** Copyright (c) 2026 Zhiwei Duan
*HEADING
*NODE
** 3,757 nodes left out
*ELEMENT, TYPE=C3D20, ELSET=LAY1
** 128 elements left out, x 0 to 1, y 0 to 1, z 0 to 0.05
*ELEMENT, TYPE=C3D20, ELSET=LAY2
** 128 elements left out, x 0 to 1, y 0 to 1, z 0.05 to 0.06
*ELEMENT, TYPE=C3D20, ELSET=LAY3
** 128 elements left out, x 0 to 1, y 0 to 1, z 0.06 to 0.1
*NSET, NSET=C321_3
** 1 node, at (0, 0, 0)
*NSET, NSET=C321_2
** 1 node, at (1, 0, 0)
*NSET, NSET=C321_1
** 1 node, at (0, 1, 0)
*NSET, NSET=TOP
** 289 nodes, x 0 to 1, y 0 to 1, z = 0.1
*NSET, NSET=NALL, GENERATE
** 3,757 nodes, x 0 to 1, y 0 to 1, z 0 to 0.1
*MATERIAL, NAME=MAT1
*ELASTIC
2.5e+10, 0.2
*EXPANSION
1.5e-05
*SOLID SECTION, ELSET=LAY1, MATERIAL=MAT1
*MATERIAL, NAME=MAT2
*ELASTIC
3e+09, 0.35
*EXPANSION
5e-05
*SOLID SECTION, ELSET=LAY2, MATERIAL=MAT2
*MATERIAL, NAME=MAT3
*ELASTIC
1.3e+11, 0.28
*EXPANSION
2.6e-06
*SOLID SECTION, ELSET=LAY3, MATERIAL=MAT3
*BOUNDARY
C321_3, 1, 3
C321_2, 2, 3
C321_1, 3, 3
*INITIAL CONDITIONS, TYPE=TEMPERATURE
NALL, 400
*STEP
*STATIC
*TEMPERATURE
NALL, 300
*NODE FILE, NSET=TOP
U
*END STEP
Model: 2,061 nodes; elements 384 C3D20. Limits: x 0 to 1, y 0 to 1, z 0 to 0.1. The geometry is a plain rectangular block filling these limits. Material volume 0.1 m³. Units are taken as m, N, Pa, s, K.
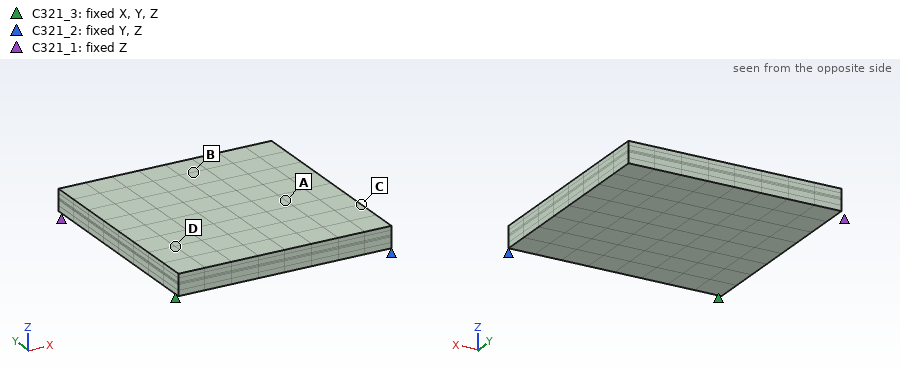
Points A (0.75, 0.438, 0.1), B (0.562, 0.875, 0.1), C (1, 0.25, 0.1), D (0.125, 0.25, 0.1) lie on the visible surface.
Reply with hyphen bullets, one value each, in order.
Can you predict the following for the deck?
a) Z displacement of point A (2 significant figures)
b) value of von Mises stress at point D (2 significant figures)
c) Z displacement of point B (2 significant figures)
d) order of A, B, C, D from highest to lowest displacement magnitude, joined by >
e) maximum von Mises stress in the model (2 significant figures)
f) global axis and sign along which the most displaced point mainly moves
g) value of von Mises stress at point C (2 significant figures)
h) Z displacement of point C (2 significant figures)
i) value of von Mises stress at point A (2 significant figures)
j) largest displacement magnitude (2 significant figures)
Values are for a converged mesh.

- 0.0035 m
- 4.7e+07 Pa
- 0.0028 m
- A > B > D > C
- 5.0e+07 Pa
- +Z
- 3.6e+07 Pa
- 0.0014 m
- 5.0e+07 Pa
- 0.0045 m
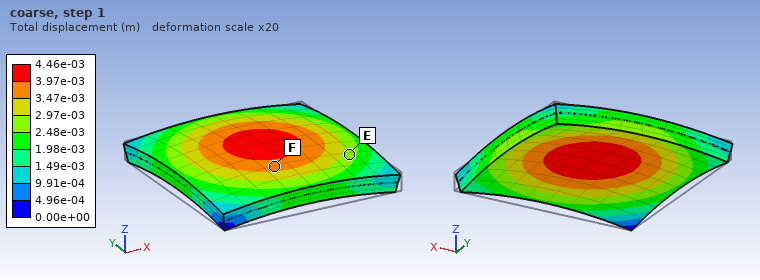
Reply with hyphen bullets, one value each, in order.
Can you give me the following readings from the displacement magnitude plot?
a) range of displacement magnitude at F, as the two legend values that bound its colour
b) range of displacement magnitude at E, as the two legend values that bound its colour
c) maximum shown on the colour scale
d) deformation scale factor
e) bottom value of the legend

- 3.47e-03 to 3.97e-03 m
- 2.48e-03 to 2.97e-03 m
- 4.46e-03 m
- 20
- 0.00e+00 m
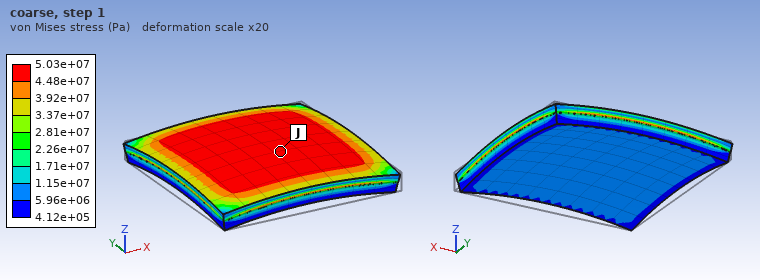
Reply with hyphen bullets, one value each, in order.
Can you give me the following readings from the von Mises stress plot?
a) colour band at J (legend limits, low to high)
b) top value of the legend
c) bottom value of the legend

- 4.48e+07 to 5.03e+07 Pa
- 5.03e+07 Pa
- 4.12e+05 Pa
